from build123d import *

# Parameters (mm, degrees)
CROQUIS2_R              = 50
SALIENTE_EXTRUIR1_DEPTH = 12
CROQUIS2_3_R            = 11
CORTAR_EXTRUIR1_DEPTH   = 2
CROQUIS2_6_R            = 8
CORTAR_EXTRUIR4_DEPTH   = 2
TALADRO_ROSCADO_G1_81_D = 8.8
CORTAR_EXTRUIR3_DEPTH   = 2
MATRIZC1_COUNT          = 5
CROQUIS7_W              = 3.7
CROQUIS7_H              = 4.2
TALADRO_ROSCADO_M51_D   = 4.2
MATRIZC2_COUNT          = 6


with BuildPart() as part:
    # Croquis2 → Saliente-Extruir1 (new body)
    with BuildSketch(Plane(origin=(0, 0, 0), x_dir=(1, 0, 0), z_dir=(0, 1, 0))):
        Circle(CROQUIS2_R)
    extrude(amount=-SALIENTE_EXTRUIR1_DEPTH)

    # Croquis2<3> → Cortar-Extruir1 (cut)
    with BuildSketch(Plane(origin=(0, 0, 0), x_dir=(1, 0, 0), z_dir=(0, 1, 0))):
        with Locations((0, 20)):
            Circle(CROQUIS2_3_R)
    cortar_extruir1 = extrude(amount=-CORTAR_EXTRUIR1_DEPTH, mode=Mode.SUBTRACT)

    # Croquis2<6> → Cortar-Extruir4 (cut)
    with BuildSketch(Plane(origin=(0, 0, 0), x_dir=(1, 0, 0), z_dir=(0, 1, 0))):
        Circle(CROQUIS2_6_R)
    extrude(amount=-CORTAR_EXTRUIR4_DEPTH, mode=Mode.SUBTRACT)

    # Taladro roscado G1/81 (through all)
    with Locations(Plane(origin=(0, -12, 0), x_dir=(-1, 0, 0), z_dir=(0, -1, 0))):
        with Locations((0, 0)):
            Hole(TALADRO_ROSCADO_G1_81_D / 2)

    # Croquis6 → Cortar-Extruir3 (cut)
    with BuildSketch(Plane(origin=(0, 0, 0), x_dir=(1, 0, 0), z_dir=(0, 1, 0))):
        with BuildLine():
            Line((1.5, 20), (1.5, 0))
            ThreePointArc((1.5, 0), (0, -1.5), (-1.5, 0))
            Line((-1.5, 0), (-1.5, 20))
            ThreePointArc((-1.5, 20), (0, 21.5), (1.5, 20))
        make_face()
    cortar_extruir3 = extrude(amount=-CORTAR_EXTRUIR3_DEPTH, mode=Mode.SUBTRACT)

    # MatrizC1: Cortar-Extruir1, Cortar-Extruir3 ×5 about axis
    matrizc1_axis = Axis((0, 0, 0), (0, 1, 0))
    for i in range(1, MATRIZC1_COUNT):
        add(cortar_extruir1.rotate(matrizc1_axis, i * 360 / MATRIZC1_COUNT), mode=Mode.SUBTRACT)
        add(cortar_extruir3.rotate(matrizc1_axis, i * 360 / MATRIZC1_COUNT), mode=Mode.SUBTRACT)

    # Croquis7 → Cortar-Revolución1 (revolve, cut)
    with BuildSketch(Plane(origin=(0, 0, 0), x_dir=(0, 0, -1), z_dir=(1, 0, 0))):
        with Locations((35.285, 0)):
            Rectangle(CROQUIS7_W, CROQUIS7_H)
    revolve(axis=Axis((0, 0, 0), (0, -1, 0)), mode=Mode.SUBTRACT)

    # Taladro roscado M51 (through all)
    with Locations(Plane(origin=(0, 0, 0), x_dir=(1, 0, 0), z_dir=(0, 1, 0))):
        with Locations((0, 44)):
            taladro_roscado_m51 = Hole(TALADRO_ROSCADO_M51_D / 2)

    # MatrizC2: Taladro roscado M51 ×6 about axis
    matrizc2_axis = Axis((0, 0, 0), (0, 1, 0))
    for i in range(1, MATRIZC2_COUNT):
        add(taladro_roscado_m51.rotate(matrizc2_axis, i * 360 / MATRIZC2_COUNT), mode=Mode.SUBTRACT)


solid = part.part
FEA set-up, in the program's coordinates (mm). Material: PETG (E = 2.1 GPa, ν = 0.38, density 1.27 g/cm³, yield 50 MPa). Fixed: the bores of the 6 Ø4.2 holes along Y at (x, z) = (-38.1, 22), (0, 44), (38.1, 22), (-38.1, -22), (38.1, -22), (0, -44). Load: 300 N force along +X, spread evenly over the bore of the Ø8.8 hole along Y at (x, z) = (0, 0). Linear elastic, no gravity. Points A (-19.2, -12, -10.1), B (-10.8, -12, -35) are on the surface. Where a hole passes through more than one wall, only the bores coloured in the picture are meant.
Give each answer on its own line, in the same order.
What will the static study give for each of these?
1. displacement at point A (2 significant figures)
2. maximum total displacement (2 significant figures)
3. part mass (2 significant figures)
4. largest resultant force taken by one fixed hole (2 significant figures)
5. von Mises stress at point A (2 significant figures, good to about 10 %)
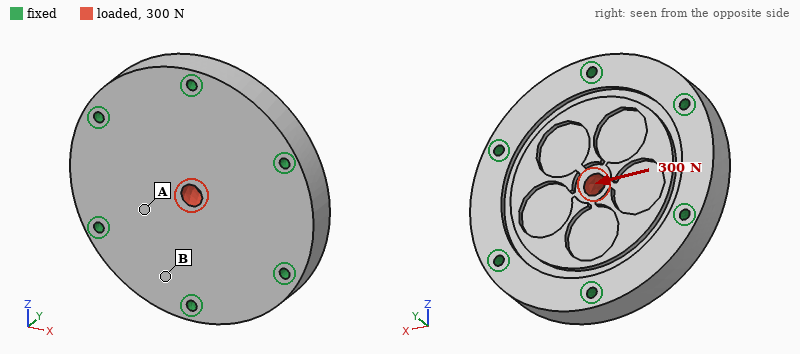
4.4 µm
11 µm
110 g
67 N
0.39 MPa
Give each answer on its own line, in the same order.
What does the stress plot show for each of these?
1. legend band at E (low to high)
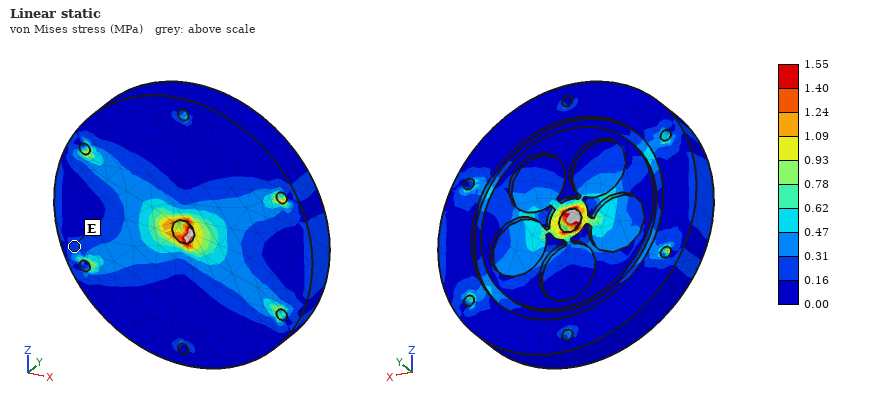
0.16 to 0.31 MPa
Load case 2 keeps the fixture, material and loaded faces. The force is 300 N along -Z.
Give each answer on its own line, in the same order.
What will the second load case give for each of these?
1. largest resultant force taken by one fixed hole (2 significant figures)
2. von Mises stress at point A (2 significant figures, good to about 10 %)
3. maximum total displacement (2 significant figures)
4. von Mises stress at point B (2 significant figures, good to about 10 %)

77 N
0.23 MPa
11 µm
0.17 MPa
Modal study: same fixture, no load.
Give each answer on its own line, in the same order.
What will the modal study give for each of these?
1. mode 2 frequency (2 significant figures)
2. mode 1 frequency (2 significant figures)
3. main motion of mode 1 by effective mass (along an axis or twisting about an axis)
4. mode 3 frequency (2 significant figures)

4500 Hz
2400 Hz
along Y
4500 Hz
